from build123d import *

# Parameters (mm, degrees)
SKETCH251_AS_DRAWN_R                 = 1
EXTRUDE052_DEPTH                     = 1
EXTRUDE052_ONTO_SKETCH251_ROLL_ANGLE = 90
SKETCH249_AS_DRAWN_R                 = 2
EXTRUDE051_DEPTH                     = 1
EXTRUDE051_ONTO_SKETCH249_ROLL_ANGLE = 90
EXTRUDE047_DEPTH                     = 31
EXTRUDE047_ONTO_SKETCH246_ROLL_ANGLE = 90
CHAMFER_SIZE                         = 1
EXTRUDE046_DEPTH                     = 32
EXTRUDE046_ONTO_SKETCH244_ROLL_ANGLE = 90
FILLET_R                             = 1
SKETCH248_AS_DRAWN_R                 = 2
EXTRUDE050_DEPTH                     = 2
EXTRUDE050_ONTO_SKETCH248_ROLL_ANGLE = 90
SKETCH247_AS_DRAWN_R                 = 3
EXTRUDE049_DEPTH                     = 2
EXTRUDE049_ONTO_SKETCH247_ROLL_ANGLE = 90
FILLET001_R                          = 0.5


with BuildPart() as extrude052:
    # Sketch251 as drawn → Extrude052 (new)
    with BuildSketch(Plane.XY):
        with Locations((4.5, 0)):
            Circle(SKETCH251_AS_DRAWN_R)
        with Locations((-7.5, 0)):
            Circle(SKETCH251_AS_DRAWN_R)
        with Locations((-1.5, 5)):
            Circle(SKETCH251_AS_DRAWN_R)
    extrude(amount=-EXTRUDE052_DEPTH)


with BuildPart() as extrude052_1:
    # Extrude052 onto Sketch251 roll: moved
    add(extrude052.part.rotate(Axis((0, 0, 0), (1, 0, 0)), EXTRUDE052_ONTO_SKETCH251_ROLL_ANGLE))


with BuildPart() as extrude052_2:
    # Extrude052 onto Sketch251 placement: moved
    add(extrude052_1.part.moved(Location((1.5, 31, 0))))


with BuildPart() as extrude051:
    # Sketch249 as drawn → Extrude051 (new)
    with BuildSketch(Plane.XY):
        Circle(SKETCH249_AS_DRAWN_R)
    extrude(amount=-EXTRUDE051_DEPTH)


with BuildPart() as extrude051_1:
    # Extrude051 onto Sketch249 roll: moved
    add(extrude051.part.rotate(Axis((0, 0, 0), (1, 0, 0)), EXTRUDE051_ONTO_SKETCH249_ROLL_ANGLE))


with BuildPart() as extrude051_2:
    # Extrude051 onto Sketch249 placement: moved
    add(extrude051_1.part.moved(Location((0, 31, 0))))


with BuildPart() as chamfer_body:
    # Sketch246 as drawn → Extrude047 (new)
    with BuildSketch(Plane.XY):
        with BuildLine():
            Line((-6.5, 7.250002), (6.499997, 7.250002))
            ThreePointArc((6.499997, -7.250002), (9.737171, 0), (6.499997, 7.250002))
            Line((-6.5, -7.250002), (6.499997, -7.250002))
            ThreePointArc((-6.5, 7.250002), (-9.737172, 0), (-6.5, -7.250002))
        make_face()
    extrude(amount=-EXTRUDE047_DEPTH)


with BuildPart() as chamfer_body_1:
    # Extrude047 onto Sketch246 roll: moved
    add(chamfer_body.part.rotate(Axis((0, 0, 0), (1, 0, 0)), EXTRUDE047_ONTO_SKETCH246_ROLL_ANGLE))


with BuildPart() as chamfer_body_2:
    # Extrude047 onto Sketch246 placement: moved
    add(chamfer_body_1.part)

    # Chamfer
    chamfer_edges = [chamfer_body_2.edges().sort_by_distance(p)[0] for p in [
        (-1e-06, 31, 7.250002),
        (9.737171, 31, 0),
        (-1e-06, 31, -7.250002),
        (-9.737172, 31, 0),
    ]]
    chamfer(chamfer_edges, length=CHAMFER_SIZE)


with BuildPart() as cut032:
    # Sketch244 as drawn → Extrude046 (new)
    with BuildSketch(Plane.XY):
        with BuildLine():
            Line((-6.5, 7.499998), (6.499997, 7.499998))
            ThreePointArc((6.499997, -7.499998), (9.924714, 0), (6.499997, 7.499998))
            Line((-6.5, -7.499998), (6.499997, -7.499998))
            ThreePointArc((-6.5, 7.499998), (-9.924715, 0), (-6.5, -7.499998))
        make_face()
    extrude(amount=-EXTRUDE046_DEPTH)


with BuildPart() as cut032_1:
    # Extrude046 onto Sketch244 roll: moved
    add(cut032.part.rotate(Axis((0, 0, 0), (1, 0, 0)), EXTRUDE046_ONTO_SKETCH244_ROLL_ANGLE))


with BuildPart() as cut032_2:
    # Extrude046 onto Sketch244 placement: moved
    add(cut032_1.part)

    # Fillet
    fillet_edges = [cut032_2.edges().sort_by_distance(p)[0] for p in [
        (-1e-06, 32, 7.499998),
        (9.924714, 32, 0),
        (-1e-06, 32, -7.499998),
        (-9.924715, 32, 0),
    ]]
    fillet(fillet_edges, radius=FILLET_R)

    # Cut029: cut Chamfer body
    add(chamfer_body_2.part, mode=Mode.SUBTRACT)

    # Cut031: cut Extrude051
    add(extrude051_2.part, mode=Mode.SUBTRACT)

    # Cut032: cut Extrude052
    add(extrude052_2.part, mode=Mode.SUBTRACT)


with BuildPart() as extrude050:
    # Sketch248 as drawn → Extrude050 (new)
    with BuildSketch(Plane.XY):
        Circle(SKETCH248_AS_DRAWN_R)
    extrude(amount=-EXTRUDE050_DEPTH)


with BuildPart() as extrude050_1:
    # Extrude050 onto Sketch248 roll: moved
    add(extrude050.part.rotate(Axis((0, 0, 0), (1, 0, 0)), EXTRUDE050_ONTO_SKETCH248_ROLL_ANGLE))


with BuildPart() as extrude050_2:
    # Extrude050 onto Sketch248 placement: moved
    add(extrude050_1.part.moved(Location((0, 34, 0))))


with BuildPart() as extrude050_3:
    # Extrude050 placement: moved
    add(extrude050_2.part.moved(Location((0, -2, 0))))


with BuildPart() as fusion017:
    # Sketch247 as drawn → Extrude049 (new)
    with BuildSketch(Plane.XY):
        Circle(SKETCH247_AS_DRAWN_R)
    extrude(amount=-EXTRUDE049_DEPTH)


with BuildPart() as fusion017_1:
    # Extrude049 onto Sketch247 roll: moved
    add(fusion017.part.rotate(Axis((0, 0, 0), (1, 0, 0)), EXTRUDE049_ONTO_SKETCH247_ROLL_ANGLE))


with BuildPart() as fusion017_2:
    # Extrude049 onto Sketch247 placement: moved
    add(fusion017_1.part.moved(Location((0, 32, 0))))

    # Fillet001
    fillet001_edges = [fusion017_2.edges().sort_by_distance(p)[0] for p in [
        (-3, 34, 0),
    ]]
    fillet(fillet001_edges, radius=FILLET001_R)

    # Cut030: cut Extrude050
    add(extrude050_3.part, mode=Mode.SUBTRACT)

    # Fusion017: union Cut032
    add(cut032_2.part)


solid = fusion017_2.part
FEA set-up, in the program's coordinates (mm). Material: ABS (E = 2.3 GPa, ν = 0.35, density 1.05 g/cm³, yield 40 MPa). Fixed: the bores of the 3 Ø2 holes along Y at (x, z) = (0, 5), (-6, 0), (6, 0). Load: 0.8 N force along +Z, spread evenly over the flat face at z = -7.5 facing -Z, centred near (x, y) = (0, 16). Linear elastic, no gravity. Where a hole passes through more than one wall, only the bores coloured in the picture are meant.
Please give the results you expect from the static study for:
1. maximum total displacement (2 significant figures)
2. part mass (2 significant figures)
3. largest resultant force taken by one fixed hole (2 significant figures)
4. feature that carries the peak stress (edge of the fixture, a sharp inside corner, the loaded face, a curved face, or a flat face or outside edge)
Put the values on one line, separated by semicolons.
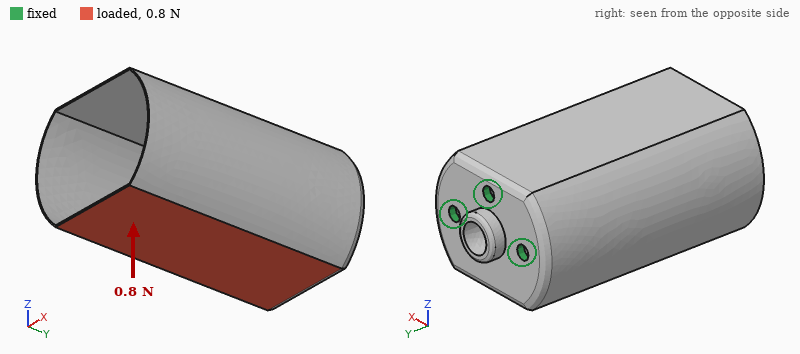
0.49 mm; 0.72 g; 1.0 N; the loaded face
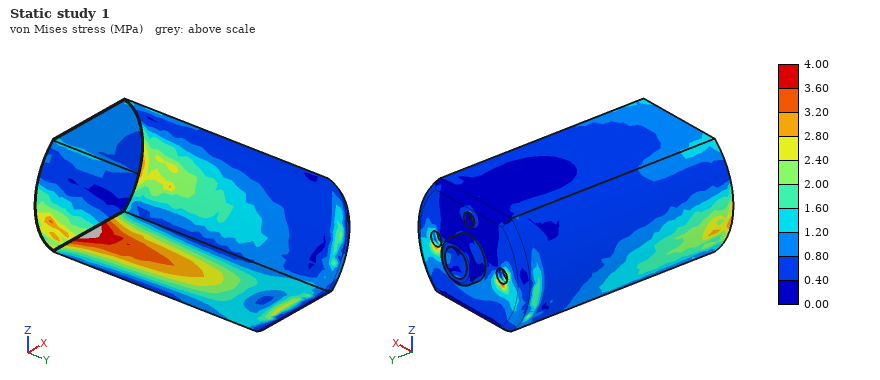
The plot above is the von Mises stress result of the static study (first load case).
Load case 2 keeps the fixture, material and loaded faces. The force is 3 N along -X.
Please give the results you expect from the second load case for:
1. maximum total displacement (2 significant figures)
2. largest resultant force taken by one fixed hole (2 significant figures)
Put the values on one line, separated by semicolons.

0.49 mm; 4.2 N
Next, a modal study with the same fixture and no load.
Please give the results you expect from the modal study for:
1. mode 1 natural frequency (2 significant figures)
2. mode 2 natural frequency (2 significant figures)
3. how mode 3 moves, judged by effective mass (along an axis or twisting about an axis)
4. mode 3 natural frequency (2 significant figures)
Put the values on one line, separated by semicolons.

640 Hz; 760 Hz; along Z; 1000 Hz
